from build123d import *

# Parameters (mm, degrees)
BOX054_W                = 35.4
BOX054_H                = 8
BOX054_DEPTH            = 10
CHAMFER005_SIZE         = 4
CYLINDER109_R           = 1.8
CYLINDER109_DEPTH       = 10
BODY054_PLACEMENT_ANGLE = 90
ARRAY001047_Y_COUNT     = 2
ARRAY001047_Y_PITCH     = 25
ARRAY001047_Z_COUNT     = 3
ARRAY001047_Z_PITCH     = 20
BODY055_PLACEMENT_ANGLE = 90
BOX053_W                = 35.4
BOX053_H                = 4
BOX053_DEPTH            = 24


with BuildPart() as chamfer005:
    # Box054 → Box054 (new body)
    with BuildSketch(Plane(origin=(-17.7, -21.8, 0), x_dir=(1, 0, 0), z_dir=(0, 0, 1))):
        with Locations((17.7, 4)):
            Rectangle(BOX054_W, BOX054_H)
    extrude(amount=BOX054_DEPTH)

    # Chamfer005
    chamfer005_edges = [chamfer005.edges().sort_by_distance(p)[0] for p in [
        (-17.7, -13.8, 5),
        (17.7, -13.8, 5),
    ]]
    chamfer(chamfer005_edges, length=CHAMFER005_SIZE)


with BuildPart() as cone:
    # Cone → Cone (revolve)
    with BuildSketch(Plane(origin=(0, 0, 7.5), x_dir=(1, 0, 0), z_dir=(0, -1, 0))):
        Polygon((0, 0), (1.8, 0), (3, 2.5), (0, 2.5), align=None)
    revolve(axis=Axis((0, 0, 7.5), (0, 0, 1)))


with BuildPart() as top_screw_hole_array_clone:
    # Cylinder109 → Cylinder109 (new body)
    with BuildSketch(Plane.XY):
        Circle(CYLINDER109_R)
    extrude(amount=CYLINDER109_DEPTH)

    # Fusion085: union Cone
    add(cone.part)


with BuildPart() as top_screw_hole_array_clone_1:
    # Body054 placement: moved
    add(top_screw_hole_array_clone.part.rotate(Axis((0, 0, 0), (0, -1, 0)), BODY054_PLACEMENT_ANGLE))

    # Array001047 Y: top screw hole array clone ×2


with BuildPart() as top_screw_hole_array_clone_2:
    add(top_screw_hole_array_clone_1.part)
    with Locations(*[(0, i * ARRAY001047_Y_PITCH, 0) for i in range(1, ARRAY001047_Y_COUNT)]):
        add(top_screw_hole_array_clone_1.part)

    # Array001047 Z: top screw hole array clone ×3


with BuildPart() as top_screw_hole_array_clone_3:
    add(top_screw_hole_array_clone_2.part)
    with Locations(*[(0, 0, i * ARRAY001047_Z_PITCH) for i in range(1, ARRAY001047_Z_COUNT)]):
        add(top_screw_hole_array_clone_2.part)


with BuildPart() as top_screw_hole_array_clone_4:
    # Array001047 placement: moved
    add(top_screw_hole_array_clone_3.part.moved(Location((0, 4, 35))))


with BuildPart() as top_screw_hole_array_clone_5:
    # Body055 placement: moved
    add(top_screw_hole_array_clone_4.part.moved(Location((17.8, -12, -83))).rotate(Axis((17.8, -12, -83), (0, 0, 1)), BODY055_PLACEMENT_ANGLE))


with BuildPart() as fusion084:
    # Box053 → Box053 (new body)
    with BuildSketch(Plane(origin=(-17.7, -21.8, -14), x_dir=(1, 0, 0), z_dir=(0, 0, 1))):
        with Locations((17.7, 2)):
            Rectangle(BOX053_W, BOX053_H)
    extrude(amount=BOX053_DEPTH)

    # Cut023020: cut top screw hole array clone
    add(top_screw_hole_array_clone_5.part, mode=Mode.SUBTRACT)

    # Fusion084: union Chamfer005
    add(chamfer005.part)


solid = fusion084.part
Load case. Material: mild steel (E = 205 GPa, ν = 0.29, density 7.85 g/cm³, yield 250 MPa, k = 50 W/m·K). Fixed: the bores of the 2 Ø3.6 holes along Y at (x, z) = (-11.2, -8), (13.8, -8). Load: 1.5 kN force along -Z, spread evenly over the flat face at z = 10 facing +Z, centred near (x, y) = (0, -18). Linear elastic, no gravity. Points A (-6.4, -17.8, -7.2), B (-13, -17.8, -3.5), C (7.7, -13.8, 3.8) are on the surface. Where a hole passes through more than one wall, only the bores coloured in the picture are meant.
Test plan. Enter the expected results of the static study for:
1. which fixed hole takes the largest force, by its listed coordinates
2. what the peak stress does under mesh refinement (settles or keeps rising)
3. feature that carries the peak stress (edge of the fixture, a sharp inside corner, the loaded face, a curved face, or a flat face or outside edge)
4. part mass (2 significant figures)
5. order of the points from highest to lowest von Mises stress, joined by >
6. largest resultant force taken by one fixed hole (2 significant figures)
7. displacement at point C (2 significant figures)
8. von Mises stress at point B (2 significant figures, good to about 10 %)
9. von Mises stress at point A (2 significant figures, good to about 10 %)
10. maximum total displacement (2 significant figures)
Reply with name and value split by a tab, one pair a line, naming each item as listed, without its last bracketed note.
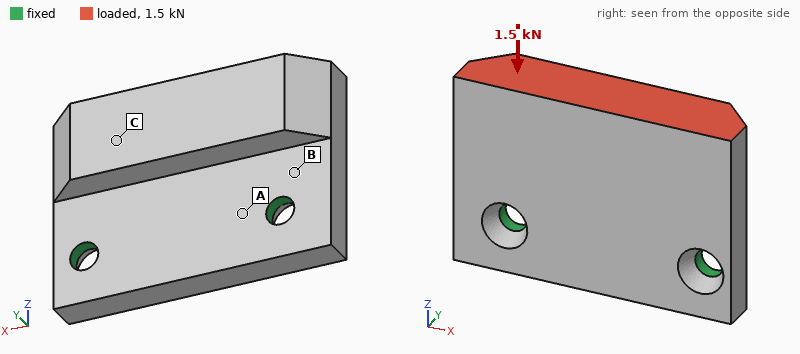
which fixed hole takes the largest force, by its listed coordinates	(-11.2, -8)
what the peak stress does under mesh refinement	keeps rising
feature that carries the peak stress	edge of the fixture
part mass	36 g
order of the points from highest to lowest von Mises stress, joined by >	B > A > C
largest resultant force taken by one fixed hole	830 N
displacement at point C	8.6 µm
von Mises stress at point B	48 MPa
von Mises stress at point A	29 MPa
maximum total displacement	13 µm
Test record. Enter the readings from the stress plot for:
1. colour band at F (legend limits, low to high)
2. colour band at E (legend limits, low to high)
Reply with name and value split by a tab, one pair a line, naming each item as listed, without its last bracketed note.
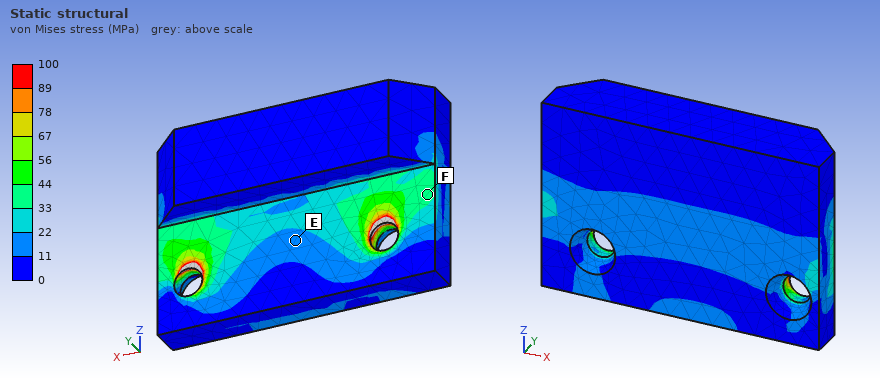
colour band at F	33 to 44 MPa
colour band at E	11 to 22 MPa
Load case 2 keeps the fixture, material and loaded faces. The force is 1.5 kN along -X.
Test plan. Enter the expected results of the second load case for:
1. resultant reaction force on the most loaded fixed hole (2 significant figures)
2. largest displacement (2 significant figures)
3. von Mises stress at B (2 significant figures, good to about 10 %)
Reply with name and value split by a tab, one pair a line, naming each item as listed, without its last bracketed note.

resultant reaction force on the most loaded fixed hole	1.3 kN
largest displacement	6.4 µm
von Mises stress at B	36 MPa
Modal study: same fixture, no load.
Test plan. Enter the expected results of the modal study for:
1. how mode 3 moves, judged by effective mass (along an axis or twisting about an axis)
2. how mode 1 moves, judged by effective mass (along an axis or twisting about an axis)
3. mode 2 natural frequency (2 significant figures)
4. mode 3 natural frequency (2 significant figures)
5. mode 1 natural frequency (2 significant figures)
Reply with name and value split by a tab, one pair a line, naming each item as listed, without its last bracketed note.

how mode 3 moves, judged by effective mass	along X
how mode 1 moves, judged by effective mass	along Y
mode 2 natural frequency	13 kHz
mode 3 natural frequency	23 kHz
mode 1 natural frequency	4700 Hz
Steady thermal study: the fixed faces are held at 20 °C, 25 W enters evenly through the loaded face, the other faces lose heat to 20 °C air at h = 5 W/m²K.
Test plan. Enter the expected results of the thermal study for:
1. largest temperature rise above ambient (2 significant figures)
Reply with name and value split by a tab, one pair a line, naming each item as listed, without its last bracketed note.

largest temperature rise above ambient	64 K
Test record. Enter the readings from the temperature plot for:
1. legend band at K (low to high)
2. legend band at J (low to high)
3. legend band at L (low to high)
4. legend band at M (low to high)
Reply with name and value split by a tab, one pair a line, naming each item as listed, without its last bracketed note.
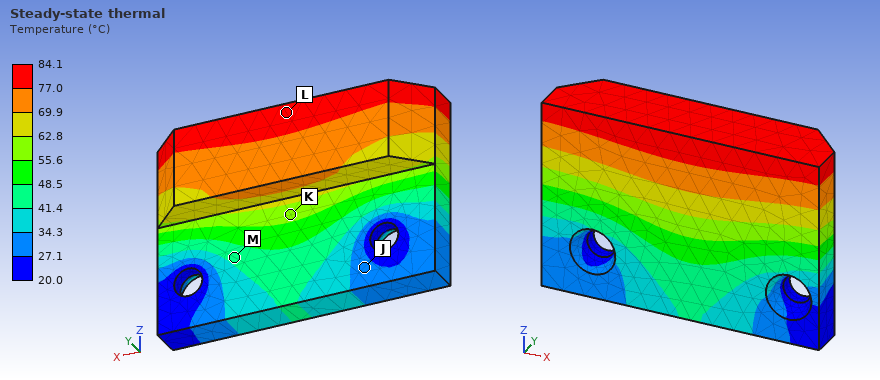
legend band at K	55.6 to 62.8 °C
legend band at J	27.1 to 34.3 °C
legend band at L	77.0 to 84.1 °C
legend band at M	41.4 to 48.5 °C
